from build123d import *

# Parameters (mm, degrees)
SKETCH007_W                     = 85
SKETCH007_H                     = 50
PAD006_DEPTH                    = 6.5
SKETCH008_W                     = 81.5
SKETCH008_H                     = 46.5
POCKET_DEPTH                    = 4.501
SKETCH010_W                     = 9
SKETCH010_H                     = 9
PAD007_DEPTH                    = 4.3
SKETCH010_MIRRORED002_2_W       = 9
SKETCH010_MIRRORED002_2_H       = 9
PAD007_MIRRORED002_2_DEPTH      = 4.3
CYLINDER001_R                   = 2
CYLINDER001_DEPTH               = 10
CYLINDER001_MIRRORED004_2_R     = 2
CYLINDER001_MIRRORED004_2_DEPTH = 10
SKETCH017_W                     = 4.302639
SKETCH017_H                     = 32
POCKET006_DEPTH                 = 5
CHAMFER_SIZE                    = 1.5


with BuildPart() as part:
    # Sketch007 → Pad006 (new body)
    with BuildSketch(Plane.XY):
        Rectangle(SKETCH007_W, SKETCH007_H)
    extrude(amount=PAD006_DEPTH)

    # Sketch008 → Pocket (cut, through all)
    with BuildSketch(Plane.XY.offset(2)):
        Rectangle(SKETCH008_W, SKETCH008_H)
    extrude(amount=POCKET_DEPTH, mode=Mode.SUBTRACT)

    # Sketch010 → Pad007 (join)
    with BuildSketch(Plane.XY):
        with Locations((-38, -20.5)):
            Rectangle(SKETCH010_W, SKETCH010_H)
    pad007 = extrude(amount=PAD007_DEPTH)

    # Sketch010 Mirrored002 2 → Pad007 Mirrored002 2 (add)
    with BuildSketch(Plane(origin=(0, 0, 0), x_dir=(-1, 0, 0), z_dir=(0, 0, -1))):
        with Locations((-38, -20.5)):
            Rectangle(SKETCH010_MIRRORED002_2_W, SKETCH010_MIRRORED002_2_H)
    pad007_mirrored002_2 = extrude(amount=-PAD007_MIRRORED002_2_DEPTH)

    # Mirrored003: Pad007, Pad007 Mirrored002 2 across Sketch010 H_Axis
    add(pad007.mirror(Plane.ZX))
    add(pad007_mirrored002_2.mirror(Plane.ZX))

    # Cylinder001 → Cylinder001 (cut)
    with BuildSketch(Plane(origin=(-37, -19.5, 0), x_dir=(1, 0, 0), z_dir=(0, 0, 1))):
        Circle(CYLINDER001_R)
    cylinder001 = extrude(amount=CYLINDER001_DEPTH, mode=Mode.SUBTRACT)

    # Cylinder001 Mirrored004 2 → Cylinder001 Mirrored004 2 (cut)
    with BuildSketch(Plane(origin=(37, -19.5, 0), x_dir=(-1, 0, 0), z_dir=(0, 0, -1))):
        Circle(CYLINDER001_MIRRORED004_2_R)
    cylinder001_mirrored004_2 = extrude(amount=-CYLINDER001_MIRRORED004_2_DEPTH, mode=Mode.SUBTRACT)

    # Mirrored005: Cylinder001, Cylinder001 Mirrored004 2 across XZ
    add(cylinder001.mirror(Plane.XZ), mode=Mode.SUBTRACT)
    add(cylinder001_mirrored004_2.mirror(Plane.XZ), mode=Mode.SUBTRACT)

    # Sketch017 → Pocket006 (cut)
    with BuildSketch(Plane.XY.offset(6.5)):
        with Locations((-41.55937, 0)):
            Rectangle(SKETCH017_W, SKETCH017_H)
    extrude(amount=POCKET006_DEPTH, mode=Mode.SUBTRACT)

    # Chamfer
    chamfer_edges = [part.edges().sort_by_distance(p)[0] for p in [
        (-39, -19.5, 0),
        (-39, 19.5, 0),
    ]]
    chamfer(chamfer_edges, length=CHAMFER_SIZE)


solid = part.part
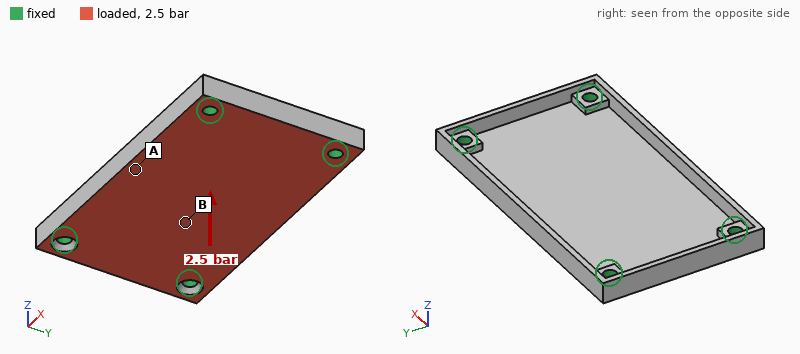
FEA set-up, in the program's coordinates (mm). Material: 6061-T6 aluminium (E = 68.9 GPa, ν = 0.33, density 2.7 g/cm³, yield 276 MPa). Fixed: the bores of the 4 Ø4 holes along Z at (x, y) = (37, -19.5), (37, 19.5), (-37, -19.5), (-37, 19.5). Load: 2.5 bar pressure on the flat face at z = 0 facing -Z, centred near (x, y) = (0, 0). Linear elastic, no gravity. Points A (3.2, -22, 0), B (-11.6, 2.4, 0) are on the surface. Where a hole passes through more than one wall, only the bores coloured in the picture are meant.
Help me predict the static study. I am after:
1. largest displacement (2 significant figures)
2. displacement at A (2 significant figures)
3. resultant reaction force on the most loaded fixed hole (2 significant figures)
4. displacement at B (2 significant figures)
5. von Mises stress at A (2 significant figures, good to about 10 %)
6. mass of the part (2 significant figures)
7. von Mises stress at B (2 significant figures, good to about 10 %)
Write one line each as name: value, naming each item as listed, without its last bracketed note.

largest displacement: 0.21 mm
displacement at A: 0.10 mm
resultant reaction force on the most loaded fixed hole: 310 N
displacement at B: 0.18 mm
von Mises stress at A: 30 MPa
mass of the part: 29 g
von Mises stress at B: 47 MPa
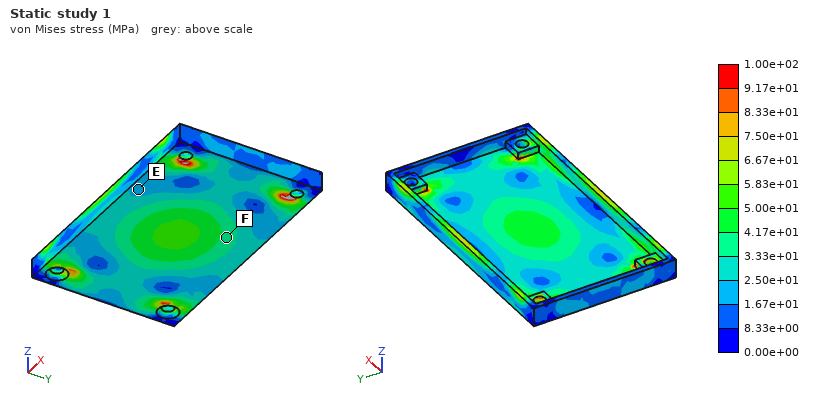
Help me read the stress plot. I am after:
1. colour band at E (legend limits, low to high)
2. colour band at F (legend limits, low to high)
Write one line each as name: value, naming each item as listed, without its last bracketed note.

colour band at E: 1.67e+01 to 2.50e+01 MPa
colour band at F: 3.33e+01 to 4.17e+01 MPa
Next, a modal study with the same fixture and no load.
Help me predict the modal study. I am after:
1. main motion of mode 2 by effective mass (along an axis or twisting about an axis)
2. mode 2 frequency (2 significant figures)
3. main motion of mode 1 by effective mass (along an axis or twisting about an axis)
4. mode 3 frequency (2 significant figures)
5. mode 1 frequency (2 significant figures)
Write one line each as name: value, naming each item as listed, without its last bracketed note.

main motion of mode 2 by effective mass: twisting about X
mode 2 frequency: 4700 Hz
main motion of mode 1 by effective mass: along Z
mode 3 frequency: 6100 Hz
mode 1 frequency: 2900 Hz
